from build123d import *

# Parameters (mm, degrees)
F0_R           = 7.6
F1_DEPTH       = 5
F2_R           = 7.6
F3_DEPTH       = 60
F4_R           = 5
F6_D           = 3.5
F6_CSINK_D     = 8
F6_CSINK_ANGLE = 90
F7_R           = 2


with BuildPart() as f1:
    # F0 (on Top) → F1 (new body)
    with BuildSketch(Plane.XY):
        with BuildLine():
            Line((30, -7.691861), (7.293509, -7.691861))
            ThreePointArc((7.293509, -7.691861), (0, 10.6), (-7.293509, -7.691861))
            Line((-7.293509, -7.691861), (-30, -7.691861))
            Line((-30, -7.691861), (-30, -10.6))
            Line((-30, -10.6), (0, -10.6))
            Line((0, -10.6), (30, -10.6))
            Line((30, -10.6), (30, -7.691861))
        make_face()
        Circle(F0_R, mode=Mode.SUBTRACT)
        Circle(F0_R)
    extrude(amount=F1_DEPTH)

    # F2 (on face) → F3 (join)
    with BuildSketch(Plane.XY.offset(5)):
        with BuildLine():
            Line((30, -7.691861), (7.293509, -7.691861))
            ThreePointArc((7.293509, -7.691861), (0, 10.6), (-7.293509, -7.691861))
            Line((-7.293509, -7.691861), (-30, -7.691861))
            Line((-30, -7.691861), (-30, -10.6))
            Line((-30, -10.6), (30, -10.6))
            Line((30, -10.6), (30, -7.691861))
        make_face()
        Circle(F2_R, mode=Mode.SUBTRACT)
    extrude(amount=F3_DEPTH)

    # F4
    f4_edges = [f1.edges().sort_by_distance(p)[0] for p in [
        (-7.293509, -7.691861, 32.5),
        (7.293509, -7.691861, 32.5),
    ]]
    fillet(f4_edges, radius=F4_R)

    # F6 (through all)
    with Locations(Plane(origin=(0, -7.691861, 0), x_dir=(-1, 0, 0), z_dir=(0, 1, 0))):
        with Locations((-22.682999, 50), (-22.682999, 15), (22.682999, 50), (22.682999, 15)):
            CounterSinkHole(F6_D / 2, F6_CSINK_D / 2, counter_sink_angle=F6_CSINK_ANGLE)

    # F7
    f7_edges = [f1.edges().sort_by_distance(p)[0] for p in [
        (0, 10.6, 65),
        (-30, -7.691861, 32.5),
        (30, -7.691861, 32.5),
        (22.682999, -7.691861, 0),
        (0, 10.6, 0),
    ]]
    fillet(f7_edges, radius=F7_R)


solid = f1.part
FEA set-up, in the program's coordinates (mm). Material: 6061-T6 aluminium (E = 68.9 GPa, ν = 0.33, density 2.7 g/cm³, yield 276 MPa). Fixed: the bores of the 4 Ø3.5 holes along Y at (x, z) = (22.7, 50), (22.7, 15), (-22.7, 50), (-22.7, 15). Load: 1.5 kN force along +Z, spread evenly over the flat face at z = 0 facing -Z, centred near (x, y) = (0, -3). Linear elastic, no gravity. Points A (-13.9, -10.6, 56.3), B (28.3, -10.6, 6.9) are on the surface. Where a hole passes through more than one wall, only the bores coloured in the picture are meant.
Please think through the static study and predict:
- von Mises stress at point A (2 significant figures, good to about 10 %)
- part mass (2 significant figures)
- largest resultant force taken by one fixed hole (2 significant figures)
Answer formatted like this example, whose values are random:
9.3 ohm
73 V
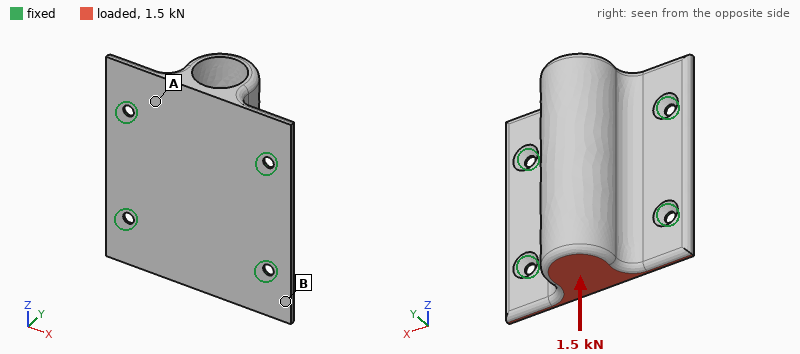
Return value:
11 MPa
61 g
470 N
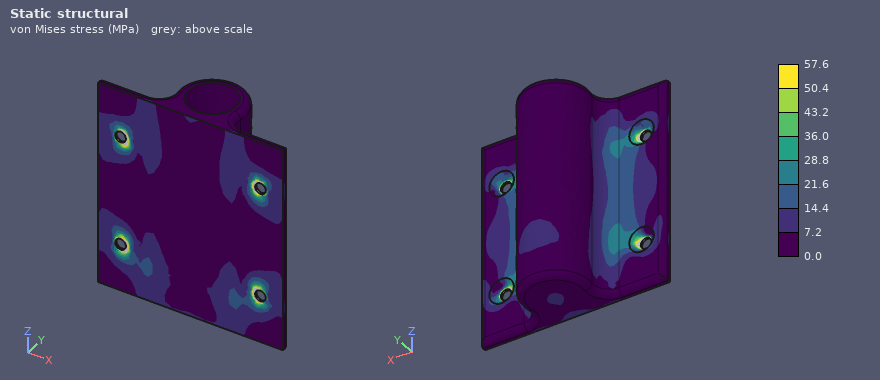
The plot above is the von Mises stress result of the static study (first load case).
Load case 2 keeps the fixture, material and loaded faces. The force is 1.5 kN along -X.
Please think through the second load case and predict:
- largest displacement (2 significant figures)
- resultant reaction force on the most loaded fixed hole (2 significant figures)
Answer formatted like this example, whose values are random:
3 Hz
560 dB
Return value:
17 µm
800 N
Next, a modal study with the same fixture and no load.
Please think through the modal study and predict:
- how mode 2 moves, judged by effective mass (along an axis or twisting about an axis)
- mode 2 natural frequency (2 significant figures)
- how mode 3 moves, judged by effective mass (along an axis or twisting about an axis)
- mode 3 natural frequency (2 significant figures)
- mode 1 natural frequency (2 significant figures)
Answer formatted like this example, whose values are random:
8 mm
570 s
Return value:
along Y
4800 Hz
along X
7900 Hz
4000 Hz
